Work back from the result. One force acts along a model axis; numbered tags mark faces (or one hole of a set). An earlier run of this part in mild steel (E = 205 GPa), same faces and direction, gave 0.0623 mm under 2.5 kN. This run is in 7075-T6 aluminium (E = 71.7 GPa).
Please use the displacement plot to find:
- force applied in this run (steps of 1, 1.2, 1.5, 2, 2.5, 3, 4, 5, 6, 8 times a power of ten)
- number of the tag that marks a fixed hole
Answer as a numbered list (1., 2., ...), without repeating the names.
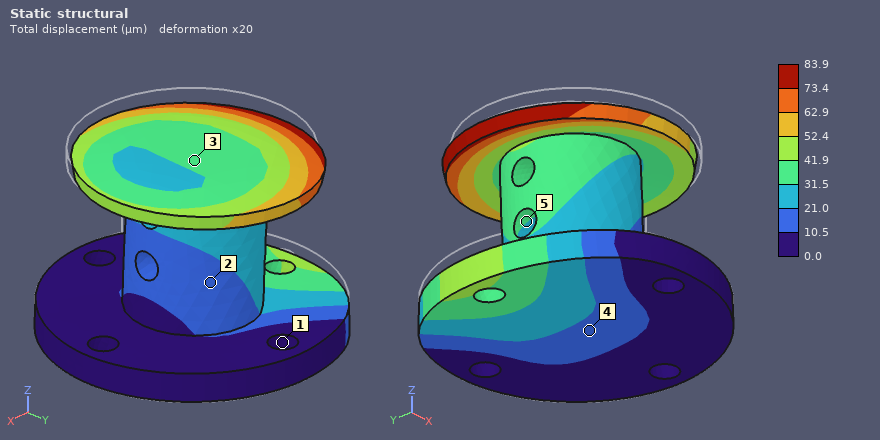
1. 1.2 kN
2. 1
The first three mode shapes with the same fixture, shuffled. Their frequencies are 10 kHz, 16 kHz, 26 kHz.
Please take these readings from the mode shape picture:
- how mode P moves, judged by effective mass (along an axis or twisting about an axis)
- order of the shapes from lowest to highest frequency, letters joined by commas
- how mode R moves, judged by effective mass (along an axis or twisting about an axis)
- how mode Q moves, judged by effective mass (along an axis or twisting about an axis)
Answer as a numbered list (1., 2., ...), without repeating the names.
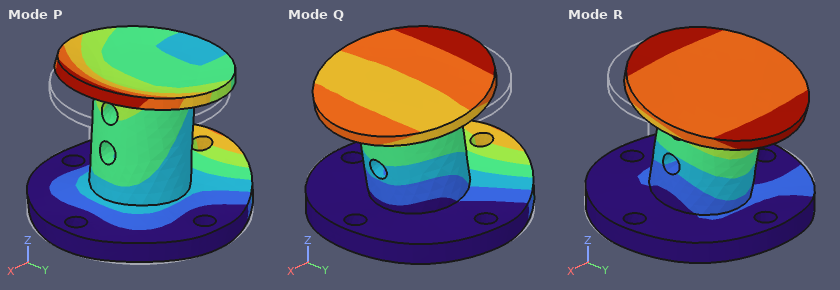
1. along Z
2. Q, R, P
3. along Y
4. along X
